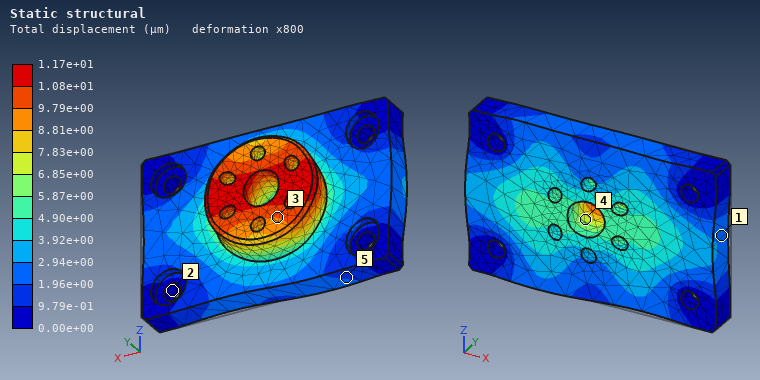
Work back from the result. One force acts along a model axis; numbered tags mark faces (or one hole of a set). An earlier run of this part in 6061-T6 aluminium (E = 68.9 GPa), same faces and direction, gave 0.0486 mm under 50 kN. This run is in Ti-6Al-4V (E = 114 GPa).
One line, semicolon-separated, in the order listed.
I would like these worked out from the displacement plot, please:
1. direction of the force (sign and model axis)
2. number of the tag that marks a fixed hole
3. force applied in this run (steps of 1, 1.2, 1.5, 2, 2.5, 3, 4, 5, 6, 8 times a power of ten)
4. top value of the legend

-X; 2; 20 kN; 1.17e+01 µm
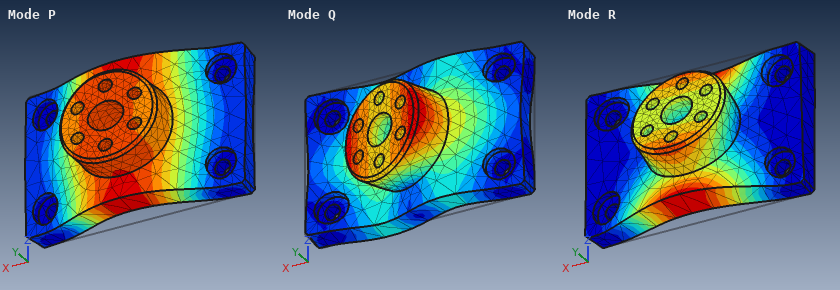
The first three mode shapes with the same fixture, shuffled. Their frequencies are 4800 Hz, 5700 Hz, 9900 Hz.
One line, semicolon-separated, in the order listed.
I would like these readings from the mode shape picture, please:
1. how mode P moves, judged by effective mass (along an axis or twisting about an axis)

along Y
